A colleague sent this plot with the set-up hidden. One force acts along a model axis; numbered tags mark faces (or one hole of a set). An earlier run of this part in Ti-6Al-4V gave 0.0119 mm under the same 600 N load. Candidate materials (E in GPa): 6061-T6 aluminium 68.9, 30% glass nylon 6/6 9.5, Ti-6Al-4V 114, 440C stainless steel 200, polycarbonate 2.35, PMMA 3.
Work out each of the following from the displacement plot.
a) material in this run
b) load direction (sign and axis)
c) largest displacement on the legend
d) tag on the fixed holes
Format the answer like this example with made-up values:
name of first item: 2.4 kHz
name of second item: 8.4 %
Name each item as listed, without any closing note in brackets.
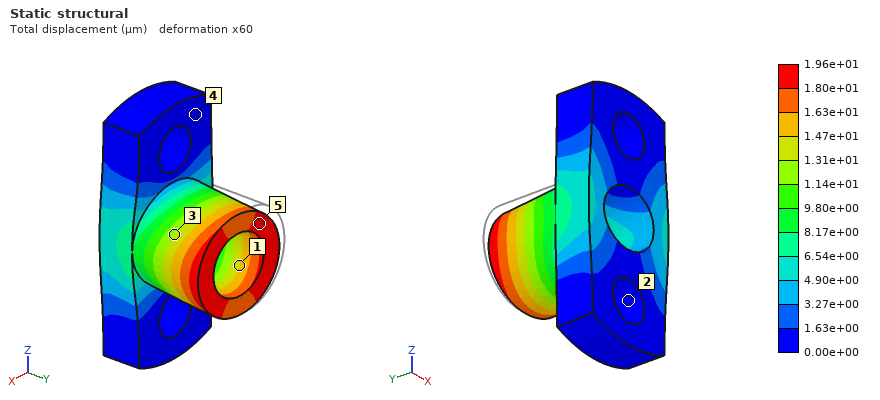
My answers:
material in this run: 6061-T6 aluminium
load direction: +X
largest displacement on the legend: 1.96e+01 µm
tag on the fixed holes: 2
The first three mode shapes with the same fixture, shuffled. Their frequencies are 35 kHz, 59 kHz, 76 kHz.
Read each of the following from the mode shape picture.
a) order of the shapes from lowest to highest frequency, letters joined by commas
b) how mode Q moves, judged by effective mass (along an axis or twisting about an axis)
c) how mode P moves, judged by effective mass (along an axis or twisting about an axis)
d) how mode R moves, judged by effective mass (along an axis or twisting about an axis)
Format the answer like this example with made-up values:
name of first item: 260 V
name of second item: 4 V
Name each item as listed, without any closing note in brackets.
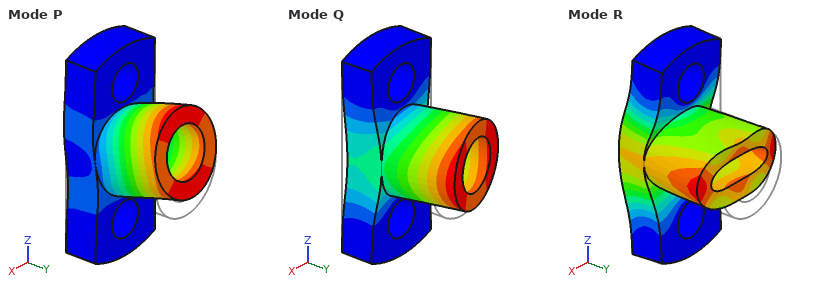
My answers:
order of the shapes from lowest to highest frequency, letters joined by commas: Q, P, R
how mode Q moves, judged by effective mass: along X
how mode P moves, judged by effective mass: along Z
how mode R moves, judged by effective mass: along Y
